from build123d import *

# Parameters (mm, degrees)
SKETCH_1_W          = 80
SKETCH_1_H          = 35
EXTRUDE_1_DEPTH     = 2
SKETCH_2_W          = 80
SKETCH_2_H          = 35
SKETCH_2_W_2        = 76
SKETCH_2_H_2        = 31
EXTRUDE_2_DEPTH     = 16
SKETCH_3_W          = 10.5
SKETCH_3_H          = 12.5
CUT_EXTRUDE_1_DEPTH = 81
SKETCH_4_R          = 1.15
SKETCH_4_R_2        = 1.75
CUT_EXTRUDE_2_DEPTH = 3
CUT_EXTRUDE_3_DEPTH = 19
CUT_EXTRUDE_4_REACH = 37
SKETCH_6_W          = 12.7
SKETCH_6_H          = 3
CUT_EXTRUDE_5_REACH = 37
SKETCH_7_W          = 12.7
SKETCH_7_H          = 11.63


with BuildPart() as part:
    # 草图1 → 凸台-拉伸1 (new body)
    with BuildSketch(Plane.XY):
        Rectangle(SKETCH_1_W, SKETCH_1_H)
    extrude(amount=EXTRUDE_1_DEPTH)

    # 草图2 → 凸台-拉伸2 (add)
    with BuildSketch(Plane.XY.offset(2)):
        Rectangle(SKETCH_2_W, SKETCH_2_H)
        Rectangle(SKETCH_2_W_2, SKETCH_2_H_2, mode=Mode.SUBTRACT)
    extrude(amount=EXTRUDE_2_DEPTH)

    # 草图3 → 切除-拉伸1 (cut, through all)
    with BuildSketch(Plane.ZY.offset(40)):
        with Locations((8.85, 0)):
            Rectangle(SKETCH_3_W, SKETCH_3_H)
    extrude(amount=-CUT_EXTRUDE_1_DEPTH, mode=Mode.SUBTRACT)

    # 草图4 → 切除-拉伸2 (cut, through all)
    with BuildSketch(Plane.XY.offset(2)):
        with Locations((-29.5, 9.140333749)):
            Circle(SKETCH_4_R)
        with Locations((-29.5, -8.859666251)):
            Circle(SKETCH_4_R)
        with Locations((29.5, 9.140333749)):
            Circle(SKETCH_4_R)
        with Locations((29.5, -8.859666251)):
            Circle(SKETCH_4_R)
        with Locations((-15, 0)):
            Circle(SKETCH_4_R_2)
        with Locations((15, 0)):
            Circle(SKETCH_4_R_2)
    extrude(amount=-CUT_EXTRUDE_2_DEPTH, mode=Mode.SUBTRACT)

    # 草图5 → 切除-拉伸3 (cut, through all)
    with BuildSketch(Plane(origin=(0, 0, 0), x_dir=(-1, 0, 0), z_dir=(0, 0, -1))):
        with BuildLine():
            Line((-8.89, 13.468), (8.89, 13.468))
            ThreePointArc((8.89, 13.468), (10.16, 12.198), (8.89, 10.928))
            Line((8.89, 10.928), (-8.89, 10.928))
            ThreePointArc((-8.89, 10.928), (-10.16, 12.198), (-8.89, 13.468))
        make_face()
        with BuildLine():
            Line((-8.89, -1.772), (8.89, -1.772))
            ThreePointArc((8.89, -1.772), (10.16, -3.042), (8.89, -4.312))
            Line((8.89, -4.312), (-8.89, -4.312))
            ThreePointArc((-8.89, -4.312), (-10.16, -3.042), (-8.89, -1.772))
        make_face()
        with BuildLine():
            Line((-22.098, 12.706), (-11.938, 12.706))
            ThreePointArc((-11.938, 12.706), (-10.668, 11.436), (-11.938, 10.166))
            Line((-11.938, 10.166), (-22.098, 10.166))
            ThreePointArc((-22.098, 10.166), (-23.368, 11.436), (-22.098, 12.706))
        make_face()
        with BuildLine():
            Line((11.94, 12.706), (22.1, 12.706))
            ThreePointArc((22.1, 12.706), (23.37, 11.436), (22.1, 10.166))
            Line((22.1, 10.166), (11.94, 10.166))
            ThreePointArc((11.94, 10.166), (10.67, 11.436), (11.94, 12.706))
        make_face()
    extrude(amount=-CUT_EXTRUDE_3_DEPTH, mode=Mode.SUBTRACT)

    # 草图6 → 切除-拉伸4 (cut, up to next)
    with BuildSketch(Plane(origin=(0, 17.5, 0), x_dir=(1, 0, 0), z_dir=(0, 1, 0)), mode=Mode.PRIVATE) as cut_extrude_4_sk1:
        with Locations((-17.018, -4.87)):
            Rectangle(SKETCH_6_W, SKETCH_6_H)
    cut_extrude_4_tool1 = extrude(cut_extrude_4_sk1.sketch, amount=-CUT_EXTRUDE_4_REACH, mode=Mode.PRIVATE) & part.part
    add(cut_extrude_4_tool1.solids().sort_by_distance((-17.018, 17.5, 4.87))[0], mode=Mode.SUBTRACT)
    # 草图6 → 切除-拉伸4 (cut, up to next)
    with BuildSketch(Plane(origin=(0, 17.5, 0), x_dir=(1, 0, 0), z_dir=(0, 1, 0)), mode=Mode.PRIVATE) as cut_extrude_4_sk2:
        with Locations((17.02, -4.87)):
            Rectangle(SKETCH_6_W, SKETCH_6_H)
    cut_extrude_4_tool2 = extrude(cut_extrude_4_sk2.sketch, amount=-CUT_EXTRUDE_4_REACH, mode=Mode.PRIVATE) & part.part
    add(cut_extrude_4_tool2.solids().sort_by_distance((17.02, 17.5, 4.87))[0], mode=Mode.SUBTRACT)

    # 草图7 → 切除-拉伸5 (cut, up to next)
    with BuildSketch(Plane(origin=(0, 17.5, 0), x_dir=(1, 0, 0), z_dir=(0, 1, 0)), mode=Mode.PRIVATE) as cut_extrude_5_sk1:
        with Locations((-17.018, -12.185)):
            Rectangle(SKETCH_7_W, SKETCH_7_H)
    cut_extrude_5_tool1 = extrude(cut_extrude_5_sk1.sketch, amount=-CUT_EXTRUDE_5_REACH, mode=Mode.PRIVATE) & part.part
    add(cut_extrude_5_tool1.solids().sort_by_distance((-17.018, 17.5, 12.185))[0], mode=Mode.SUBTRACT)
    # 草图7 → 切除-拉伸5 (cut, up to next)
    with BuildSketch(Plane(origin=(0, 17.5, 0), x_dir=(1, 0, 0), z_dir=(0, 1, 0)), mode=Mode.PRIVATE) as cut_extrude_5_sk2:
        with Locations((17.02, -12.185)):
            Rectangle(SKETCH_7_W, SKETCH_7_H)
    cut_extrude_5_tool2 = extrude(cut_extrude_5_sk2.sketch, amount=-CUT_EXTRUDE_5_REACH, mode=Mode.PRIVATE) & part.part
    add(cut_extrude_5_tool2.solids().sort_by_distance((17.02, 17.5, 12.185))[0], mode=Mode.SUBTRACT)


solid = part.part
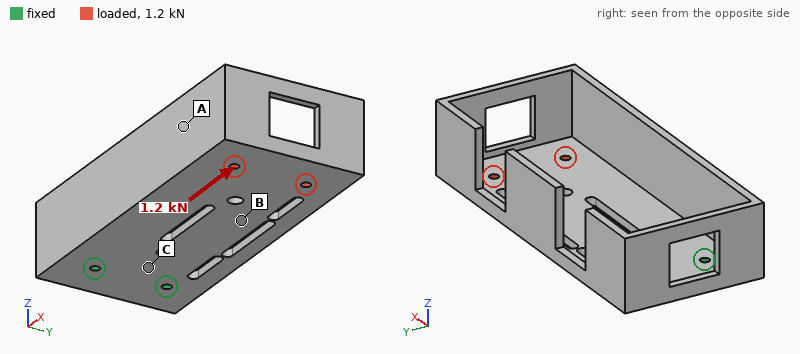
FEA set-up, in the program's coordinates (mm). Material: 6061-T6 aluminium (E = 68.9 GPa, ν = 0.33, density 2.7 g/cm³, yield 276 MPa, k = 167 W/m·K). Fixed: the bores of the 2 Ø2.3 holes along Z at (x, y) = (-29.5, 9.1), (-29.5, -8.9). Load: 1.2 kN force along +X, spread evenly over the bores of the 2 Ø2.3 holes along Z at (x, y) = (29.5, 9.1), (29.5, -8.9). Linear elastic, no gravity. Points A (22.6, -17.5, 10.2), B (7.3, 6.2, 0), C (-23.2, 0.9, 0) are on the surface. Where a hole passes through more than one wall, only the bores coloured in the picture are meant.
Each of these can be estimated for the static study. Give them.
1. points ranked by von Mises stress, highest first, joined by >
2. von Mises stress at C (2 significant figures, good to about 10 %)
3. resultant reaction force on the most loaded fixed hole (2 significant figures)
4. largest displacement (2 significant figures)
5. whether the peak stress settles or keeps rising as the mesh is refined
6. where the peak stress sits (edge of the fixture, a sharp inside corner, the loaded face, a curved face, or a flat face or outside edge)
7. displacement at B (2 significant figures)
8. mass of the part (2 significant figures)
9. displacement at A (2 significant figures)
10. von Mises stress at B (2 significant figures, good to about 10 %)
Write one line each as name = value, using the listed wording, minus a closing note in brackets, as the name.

points ranked by von Mises stress, highest first, joined by > = B > C > A
von Mises stress at C = 12 MPa
resultant reaction force on the most loaded fixed hole = 600 N
largest displacement = 55 µm
whether the peak stress settles or keeps rising as the mesh is refined = keeps rising
where the peak stress sits = edge of the fixture
displacement at B = 17 µm
mass of the part = 30 g
displacement at A = 26 µm
von Mises stress at B = 22 MPa
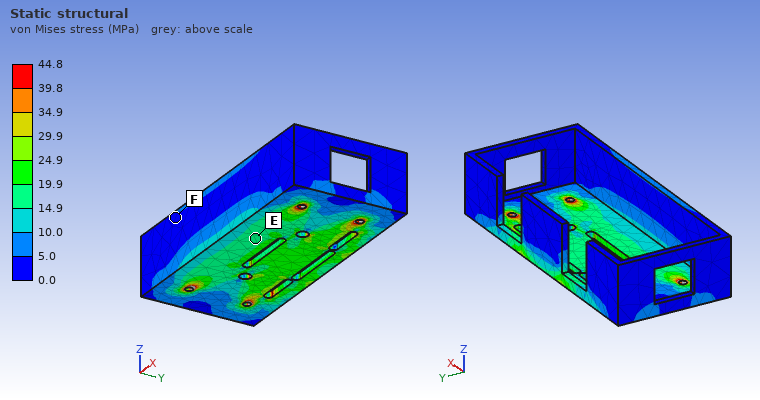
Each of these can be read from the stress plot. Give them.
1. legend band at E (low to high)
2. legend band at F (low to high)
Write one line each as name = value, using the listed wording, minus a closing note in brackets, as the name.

legend band at E = 14.9 to 19.9 MPa
legend band at F = 0.0 to 5.0 MPa
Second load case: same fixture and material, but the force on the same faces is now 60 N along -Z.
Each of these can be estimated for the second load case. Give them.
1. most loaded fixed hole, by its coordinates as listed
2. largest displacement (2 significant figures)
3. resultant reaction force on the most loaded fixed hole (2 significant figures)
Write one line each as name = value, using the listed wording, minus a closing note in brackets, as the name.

most loaded fixed hole, by its coordinates as listed = (-29.5, -8.9)
largest displacement = 0.84 mm
resultant reaction force on the most loaded fixed hole = 34 N
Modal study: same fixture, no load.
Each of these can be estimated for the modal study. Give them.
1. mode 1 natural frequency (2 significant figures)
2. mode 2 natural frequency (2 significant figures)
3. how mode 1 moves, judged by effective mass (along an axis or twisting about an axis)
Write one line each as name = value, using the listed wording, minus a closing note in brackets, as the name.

mode 1 natural frequency = 430 Hz
mode 2 natural frequency = 900 Hz
how mode 1 moves, judged by effective mass = along Z
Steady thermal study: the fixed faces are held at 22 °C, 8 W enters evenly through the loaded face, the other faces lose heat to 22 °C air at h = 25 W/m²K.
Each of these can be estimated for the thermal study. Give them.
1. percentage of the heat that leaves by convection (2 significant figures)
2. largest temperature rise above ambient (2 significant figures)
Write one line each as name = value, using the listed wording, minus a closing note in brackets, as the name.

percentage of the heat that leaves by convection = 42 %
largest temperature rise above ambient = 25 K
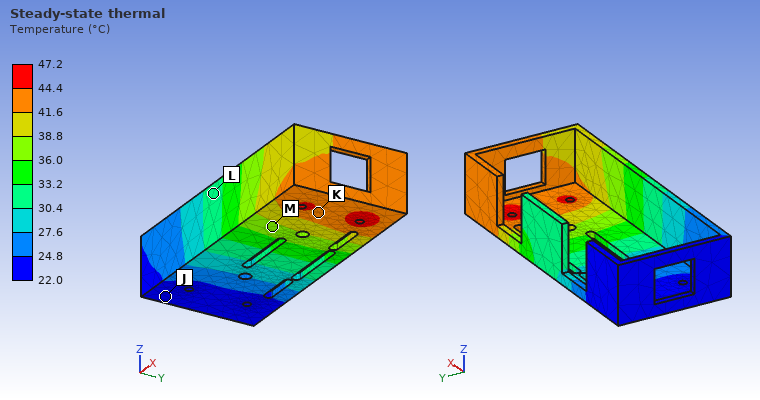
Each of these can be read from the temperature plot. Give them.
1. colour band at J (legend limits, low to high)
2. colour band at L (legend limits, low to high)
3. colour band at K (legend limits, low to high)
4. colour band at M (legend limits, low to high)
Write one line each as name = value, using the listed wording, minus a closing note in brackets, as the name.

colour band at J = 22.0 to 24.8 °C
colour band at L = 30.4 to 33.2 °C
colour band at K = 41.6 to 44.4 °C
colour band at M = 36.0 to 38.8 °C
